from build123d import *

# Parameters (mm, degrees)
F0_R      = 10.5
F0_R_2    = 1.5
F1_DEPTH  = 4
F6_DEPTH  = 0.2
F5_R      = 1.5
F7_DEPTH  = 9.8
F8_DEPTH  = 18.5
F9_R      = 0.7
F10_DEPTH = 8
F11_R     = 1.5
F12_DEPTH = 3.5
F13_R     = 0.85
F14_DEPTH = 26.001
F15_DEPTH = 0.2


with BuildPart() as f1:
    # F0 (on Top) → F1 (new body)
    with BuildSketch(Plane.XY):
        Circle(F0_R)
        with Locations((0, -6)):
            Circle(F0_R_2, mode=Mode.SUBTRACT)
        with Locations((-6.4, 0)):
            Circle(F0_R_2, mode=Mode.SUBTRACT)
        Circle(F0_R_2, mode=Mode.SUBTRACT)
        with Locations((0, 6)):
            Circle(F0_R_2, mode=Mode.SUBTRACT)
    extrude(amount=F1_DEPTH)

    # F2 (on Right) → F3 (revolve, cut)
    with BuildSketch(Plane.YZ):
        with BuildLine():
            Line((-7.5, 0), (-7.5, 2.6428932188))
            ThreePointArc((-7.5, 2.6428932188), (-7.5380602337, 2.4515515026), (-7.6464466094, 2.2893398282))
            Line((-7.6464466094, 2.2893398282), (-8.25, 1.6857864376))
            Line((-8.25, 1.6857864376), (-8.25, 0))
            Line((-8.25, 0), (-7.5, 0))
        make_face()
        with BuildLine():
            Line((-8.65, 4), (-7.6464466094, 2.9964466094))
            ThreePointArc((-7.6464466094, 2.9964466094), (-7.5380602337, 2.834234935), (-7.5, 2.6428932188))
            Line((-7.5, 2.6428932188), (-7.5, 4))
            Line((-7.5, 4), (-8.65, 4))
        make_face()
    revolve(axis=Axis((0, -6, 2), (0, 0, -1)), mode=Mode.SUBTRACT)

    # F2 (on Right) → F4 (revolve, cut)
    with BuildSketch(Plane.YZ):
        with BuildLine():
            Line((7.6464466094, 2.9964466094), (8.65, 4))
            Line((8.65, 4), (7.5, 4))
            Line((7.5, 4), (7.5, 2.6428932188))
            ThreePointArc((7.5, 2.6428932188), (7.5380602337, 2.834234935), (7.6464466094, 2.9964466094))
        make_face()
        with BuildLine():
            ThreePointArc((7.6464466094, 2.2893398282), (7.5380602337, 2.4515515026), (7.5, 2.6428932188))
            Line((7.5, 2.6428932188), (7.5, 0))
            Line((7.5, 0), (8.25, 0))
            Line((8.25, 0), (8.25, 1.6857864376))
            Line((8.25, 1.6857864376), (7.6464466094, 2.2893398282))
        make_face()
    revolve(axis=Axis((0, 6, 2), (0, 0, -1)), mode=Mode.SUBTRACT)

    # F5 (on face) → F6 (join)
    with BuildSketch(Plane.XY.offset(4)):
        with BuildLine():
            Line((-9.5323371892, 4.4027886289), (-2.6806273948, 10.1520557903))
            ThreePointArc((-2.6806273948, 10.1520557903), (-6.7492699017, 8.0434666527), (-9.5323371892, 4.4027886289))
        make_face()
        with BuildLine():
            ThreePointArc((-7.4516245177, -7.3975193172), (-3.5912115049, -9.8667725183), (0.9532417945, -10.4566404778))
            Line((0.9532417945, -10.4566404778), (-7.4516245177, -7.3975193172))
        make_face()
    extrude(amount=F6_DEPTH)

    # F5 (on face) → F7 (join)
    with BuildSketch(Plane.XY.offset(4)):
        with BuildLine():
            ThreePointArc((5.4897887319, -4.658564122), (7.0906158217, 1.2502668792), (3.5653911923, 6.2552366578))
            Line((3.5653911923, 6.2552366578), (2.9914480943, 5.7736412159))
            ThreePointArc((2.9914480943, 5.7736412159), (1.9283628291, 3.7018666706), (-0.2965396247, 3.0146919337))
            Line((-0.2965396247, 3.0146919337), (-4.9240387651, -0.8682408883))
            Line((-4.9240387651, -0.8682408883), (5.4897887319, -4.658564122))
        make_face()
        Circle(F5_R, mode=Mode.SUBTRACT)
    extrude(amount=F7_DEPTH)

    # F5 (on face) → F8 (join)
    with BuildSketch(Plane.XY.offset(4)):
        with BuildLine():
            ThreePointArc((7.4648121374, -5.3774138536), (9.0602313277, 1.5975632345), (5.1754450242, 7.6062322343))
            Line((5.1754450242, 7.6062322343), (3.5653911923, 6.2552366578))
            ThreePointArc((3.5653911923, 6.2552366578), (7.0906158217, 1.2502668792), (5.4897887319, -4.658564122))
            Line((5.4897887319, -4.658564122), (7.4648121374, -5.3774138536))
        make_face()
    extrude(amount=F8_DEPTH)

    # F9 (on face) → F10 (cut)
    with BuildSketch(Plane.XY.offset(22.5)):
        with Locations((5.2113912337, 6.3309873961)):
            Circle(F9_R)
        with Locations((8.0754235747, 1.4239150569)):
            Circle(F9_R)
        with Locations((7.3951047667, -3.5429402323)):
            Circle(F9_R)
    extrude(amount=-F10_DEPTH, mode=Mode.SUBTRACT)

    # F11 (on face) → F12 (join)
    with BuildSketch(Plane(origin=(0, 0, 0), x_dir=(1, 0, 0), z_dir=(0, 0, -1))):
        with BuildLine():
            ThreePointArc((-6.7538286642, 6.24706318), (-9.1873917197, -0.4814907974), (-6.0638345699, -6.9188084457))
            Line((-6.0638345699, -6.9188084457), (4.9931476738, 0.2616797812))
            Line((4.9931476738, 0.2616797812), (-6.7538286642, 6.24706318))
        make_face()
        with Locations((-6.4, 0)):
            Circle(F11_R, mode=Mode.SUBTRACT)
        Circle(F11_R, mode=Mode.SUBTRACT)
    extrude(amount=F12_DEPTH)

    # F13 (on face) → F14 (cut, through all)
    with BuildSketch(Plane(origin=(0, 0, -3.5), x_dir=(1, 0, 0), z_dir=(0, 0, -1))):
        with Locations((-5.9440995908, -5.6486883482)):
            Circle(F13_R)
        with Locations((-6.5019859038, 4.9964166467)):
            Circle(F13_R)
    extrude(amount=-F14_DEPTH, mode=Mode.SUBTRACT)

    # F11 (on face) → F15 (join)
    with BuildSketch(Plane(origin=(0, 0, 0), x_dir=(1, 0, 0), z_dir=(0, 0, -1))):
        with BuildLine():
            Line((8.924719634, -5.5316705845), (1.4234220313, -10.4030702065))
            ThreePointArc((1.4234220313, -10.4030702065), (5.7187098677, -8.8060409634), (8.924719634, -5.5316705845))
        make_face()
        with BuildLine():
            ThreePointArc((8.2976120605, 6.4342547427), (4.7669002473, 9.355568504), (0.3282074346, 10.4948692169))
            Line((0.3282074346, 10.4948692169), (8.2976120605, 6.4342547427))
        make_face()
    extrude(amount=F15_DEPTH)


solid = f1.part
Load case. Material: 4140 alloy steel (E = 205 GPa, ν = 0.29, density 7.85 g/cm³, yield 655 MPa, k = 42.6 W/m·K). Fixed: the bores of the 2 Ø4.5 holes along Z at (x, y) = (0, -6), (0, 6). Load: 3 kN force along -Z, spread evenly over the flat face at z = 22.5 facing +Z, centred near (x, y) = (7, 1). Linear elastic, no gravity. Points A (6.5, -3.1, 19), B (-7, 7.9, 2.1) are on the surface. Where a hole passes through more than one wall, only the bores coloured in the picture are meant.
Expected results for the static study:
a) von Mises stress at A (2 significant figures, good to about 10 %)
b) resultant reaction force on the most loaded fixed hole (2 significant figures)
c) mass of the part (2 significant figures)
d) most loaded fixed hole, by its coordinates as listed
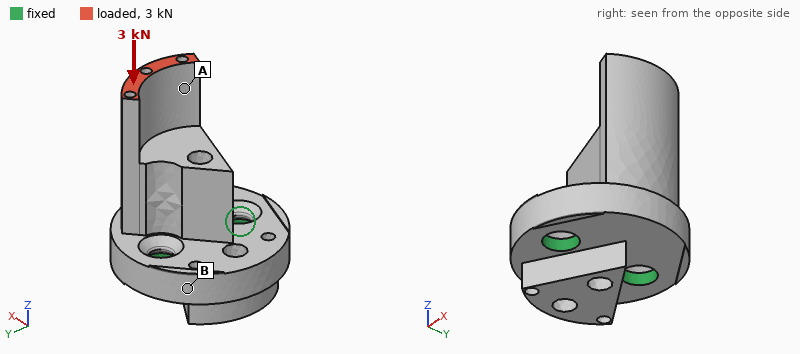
130 MPa
1.9 kN
20 g
(0, 6)
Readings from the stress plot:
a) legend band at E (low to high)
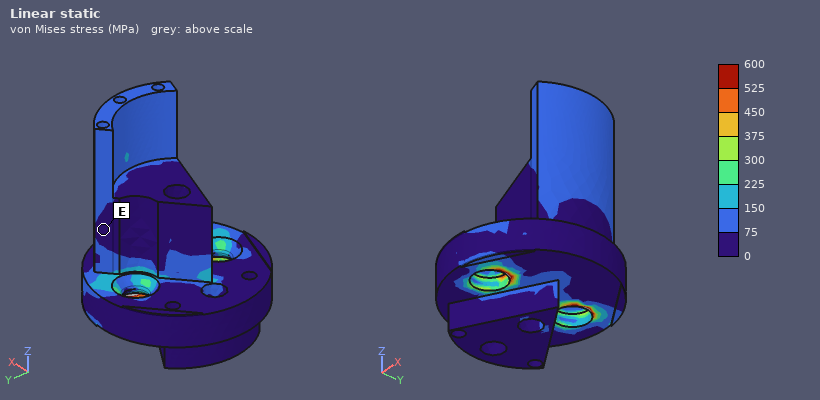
0 to 75 MPa
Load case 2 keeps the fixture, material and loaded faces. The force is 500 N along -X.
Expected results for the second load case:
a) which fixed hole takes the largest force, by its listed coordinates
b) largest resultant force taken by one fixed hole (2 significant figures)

(0, 6)
320 N
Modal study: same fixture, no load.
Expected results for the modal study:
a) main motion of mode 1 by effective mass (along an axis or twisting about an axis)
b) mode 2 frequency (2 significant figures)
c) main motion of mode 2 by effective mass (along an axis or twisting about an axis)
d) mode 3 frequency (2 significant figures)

along X
20 kHz
along Y
27 kHz
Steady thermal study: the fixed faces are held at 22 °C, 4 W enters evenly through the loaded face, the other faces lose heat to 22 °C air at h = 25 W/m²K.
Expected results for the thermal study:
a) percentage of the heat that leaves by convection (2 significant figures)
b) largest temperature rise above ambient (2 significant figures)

13 %
52 K
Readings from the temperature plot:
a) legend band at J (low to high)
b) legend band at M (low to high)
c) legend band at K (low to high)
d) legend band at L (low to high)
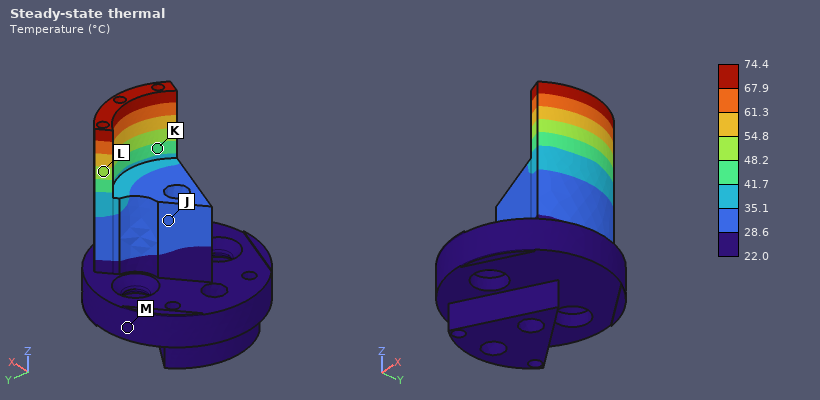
28.6 to 35.1 °C
22.0 to 28.6 °C
41.7 to 48.2 °C
48.2 to 54.8 °C
